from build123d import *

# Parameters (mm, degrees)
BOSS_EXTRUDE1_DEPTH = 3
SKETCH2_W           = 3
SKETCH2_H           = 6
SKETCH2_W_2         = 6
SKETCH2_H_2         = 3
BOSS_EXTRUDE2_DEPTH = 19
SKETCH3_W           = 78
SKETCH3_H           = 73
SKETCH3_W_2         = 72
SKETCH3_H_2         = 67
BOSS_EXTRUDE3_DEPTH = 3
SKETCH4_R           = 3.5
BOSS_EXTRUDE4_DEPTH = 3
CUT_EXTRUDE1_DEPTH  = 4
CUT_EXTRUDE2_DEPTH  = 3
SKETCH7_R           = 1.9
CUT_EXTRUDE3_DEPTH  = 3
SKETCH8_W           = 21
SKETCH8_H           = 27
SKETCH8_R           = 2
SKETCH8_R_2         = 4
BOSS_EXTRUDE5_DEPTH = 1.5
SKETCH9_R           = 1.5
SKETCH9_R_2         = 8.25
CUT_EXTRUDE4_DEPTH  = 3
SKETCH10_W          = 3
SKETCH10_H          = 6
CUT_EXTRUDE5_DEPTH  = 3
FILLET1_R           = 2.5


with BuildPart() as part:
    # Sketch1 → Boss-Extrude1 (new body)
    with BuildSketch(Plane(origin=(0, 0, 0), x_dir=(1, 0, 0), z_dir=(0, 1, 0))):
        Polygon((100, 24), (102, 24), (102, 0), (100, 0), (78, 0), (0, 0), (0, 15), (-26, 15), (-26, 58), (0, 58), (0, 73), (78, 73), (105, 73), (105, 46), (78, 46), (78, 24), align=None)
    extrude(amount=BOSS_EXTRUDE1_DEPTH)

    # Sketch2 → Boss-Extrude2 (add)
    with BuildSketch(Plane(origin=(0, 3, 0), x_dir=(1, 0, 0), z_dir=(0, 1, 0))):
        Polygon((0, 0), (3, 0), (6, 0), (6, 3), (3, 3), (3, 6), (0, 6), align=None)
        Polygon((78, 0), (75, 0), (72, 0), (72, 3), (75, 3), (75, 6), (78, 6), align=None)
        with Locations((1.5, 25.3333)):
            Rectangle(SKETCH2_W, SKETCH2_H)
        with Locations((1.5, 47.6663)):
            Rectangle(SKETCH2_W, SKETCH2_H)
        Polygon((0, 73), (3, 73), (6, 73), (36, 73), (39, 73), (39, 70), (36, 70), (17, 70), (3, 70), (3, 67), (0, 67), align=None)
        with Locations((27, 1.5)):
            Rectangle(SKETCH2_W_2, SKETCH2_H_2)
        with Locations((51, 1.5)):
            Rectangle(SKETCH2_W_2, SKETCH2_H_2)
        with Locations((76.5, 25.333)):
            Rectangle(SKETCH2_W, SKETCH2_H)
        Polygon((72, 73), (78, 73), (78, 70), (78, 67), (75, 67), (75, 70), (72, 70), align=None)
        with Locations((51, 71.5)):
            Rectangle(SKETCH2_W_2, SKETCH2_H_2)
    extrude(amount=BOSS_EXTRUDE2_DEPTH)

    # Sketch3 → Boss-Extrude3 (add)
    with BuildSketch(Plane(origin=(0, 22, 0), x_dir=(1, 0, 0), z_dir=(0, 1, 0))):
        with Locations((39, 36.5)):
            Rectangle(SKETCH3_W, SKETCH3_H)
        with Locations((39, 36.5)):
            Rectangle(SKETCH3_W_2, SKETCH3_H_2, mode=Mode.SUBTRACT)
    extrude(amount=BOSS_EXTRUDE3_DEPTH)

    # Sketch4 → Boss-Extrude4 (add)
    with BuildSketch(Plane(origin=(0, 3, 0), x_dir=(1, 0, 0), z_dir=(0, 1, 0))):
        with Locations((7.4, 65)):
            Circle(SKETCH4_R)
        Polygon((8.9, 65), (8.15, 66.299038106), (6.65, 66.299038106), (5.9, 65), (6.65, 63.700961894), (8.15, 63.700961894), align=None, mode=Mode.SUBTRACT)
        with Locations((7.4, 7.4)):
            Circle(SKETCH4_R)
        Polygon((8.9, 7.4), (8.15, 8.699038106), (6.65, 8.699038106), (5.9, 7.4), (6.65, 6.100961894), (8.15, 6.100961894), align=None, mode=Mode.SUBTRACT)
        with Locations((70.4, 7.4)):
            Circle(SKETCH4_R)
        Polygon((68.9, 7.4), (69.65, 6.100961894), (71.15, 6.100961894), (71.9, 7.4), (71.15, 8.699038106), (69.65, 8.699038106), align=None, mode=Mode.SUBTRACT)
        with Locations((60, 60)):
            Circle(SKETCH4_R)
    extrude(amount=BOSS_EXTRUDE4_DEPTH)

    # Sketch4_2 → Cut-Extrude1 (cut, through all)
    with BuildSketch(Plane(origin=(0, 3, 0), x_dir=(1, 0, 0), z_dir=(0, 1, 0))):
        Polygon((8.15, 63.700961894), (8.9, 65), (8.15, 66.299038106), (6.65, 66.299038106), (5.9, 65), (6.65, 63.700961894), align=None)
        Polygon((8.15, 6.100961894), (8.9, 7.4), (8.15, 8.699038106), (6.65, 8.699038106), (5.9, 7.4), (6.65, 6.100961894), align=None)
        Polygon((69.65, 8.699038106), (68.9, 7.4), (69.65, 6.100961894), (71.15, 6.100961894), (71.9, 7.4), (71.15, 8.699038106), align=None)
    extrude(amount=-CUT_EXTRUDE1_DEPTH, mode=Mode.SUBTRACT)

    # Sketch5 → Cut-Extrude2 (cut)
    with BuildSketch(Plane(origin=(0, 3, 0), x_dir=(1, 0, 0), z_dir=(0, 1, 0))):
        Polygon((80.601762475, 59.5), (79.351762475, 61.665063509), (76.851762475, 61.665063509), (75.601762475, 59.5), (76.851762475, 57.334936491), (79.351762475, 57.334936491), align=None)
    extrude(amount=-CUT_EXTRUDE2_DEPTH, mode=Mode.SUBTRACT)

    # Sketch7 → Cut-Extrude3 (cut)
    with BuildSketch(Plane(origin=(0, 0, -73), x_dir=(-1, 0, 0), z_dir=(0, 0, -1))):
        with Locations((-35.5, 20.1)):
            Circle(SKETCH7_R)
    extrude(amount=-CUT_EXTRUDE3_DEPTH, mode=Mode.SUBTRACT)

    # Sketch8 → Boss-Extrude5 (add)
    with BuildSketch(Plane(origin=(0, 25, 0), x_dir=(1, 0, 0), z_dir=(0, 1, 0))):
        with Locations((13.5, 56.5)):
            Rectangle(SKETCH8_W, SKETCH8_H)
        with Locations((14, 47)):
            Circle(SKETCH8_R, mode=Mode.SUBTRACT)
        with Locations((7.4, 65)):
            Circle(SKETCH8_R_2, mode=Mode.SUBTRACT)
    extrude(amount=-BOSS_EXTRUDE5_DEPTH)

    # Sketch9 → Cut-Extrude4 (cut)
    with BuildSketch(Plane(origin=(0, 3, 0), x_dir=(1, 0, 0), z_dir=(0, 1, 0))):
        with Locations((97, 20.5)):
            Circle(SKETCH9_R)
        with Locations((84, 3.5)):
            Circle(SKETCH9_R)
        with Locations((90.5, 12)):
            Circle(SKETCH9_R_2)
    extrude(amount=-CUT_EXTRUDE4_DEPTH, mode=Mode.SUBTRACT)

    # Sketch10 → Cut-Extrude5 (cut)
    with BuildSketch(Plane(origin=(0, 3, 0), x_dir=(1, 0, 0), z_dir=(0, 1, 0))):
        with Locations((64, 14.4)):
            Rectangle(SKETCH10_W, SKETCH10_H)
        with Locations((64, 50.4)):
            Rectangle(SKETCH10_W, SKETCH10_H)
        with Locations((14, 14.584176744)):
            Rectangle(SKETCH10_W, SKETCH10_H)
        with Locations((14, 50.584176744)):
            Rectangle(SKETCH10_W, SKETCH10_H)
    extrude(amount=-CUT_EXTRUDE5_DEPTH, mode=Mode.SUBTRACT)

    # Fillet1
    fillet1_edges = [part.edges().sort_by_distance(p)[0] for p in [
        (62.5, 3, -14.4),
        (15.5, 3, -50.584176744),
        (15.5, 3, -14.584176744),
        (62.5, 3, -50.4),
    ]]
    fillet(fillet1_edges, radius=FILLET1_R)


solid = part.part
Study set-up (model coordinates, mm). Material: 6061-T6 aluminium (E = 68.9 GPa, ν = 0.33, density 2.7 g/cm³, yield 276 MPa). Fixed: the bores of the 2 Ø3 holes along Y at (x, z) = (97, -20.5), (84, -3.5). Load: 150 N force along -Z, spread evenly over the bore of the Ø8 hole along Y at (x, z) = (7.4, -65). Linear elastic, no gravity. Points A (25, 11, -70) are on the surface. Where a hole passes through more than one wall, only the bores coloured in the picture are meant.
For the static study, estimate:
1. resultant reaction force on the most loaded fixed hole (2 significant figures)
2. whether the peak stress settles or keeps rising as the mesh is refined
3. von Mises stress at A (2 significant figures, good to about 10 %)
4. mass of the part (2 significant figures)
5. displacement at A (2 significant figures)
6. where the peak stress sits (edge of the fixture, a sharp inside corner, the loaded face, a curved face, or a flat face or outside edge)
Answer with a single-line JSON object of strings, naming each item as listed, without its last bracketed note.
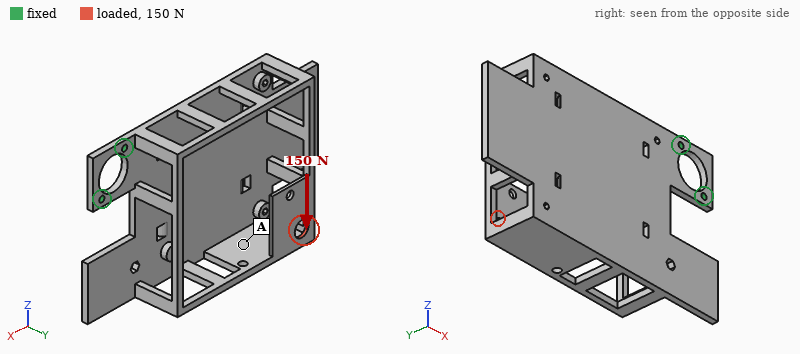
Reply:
{"resultant reaction force on the most loaded fixed hole": "590 N", "whether the peak stress settles or keeps rising as the mesh is refined": "keeps rising", "von Mises stress at A": "14 MPa", "mass of the part": "89 g", "displacement at A": "1.1 mm", "where the peak stress sits": "edge of the fixture"}
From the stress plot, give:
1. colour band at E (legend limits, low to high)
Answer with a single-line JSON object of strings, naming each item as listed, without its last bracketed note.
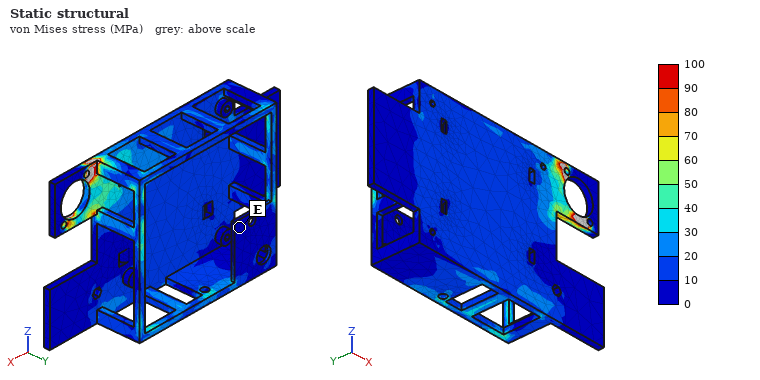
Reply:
{"colour band at E": "0 to 10 MPa"}
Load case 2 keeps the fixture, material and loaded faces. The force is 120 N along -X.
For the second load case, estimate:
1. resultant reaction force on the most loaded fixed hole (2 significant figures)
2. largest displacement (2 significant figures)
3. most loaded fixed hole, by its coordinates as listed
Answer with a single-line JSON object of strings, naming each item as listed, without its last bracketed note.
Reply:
{"resultant reaction force on the most loaded fixed hole": "380 N", "largest displacement": "1.8 mm", "most loaded fixed hole, by its coordinates as listed": "(97, -20.5)"}
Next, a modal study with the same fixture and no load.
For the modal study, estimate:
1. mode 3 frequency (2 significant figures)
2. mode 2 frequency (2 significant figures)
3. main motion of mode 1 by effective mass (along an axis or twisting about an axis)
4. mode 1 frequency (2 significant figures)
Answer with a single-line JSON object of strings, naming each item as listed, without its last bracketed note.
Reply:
{"mode 3 frequency": "730 Hz", "mode 2 frequency": "370 Hz", "main motion of mode 1 by effective mass": "along Y", "mode 1 frequency": "120 Hz"}
